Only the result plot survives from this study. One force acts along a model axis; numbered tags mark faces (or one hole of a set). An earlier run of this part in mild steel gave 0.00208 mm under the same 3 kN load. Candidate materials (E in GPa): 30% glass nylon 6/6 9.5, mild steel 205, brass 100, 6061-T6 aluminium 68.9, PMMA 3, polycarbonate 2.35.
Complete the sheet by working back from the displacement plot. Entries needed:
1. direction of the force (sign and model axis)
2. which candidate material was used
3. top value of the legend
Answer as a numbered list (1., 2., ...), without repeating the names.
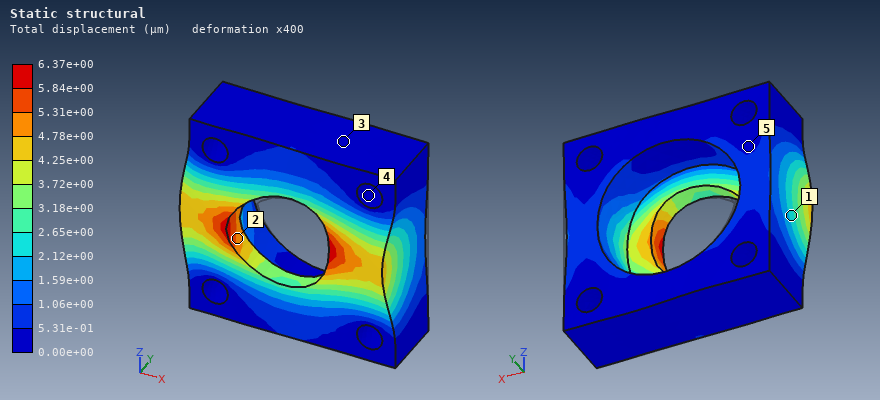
1. -X
2. 6061-T6 aluminium
3. 6.37e+00 µm
